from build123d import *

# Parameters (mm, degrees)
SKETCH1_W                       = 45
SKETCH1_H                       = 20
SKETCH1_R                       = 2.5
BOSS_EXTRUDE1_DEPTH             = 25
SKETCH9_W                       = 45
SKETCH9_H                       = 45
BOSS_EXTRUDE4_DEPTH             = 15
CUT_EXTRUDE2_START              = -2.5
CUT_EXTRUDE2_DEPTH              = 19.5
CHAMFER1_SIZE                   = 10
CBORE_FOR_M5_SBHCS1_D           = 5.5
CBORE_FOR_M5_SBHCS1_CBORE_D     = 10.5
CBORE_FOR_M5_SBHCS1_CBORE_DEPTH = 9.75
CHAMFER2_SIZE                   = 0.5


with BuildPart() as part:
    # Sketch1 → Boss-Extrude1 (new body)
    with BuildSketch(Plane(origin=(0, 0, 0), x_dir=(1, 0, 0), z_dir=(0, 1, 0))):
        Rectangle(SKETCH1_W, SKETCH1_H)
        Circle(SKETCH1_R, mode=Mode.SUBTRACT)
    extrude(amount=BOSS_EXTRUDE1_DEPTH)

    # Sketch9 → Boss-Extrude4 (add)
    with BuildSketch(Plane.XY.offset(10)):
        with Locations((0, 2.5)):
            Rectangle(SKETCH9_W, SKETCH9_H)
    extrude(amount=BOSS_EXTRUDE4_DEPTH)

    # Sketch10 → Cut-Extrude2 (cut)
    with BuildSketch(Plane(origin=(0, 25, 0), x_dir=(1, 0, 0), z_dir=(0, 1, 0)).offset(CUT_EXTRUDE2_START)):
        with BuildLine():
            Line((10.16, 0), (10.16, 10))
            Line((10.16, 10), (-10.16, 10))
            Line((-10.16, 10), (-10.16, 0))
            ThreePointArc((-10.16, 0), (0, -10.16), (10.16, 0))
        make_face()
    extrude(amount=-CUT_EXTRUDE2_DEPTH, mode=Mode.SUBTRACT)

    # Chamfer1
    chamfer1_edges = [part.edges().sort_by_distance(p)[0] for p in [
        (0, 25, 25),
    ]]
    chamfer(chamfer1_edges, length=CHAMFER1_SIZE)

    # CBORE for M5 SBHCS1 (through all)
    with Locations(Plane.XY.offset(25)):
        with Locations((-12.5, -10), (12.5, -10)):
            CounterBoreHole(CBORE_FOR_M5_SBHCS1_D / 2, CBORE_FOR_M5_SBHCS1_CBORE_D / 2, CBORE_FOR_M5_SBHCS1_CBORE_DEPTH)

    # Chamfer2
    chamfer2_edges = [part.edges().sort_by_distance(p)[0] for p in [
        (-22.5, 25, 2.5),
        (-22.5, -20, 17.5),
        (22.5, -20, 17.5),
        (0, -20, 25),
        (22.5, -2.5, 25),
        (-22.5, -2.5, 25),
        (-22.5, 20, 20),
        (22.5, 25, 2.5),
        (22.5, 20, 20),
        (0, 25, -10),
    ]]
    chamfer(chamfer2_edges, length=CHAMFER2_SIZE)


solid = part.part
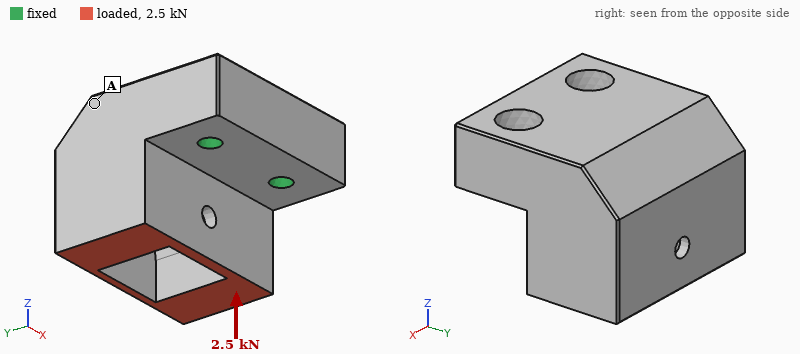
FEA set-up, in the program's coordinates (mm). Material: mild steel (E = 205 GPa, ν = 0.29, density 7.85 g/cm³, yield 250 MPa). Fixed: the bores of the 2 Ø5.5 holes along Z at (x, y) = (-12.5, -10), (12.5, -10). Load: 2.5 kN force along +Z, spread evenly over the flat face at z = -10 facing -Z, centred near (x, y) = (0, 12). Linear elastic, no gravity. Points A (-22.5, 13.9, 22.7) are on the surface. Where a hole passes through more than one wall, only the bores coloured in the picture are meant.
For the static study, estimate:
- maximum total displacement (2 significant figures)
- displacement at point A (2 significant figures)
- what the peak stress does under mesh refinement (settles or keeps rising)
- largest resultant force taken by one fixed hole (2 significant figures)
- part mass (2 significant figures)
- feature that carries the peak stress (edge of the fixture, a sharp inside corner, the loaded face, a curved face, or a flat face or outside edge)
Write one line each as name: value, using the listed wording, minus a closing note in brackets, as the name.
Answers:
maximum total displacement: 48 µm
displacement at point A: 29 µm
what the peak stress does under mesh refinement: keeps rising
largest resultant force taken by one fixed hole: 1.3 kN
part mass: 330 g
feature that carries the peak stress: edge of the fixture
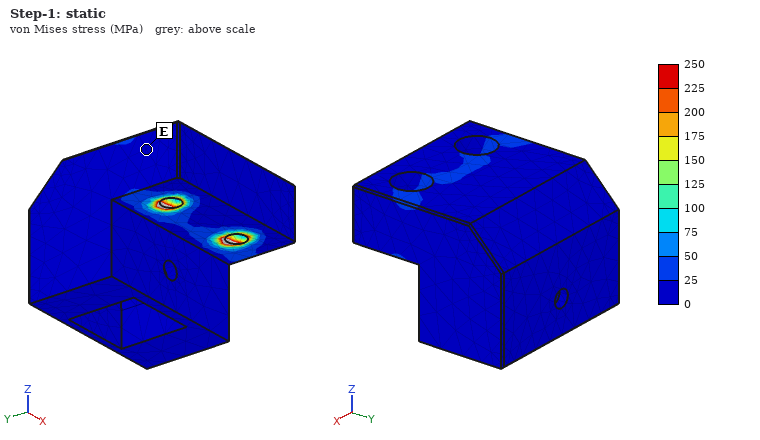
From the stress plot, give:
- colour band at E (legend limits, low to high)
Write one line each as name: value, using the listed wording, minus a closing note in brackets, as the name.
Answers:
colour band at E: 0 to 25 MPa
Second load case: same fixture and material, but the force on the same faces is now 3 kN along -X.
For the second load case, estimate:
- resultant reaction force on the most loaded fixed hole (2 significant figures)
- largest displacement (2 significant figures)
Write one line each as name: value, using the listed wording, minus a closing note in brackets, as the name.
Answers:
resultant reaction force on the most loaded fixed hole: 3.5 kN
largest displacement: 25 µm
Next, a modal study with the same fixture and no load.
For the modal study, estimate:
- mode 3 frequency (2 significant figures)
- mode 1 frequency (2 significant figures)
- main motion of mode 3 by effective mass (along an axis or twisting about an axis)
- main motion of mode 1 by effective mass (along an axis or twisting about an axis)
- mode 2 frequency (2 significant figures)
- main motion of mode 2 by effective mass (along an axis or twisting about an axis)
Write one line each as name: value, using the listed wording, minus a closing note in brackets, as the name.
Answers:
mode 3 frequency: 9800 Hz
mode 1 frequency: 2800 Hz
main motion of mode 3 by effective mass: along X
main motion of mode 1 by effective mass: along Z
mode 2 frequency: 6400 Hz
main motion of mode 2 by effective mass: along X
